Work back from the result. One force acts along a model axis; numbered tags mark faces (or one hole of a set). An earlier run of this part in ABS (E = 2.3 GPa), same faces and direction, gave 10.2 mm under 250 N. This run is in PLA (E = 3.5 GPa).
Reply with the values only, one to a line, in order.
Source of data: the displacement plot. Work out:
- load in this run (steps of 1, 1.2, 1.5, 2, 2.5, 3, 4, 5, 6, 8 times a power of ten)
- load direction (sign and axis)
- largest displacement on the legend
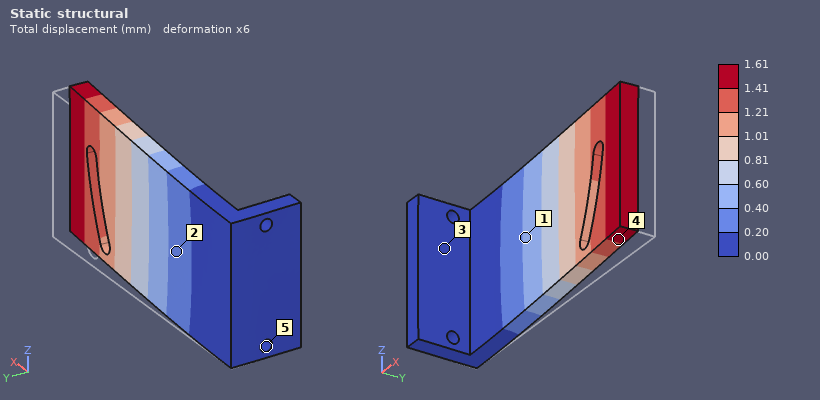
60 N
-Y
1.61 mm
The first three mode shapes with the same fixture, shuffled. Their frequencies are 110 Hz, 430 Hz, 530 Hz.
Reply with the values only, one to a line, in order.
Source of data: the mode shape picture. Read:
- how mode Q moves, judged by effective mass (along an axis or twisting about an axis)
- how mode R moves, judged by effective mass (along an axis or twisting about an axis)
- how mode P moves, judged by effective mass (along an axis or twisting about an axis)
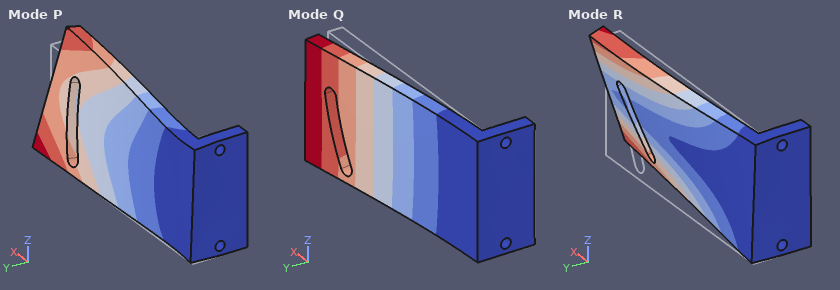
along Y
along Z
along Z
